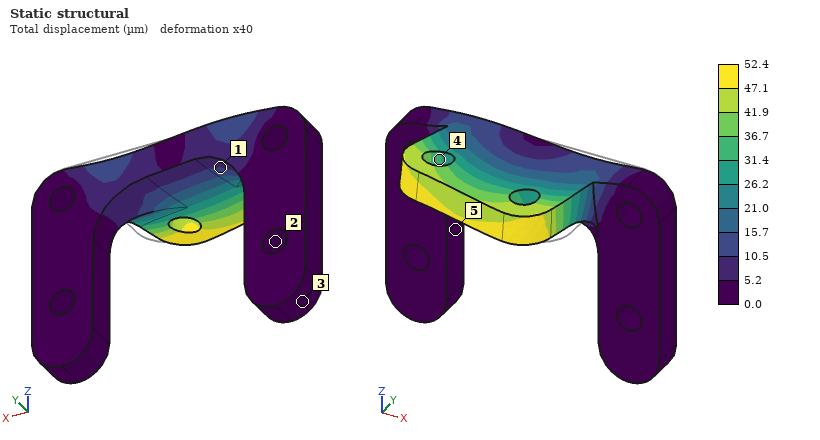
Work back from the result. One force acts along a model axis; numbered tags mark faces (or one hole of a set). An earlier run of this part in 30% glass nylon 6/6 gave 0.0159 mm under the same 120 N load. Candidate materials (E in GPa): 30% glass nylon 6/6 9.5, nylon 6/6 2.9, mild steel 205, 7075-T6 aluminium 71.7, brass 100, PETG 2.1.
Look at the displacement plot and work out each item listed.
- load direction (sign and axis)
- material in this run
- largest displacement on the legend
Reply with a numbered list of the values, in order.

1. -X
2. nylon 6/6
3. 52.4 µm
